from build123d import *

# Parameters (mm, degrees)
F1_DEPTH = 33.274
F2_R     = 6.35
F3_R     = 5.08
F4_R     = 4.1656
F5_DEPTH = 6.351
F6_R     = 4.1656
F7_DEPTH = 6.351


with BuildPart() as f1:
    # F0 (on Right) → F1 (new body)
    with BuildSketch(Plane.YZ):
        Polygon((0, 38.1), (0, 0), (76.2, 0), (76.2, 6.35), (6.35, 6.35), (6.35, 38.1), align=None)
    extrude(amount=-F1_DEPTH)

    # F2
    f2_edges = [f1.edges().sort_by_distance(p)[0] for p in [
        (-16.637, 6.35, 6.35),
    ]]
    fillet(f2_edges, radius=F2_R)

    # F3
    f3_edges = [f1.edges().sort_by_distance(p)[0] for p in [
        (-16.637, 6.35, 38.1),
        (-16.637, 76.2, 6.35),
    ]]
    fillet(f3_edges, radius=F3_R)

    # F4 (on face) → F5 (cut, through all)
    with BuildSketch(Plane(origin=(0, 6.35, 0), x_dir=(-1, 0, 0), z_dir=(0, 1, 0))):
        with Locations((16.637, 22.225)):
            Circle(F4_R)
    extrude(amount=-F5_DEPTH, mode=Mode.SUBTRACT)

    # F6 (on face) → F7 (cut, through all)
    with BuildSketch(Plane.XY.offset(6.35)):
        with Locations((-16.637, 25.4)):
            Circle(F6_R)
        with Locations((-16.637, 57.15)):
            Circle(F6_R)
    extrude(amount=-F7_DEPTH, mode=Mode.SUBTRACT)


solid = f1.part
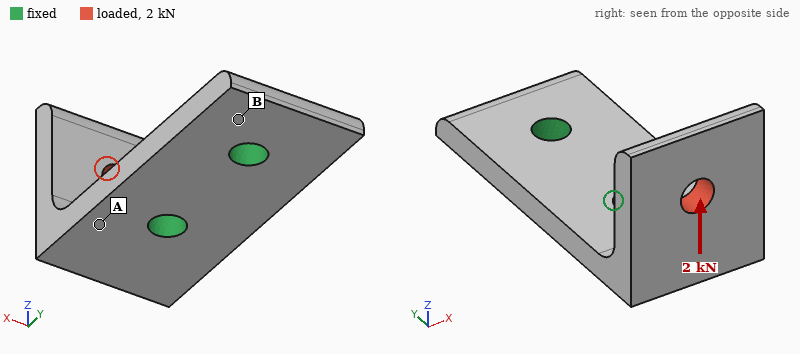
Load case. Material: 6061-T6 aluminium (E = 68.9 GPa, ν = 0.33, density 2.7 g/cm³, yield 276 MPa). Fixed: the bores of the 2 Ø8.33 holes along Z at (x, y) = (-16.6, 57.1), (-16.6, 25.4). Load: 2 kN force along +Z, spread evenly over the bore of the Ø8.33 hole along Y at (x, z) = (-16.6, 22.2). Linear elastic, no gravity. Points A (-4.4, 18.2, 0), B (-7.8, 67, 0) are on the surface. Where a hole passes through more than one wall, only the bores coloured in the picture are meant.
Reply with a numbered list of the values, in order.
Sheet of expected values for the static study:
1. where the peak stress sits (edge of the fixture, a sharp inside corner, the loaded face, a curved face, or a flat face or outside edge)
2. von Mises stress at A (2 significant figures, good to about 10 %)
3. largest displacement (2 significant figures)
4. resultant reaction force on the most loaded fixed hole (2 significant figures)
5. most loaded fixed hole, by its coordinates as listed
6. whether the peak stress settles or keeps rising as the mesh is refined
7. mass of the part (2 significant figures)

1. edge of the fixture
2. 95 MPa
3. 0.34 mm
4. 2.2 kN
5. (-16.6, 25.4)
6. keeps rising
7. 59 g
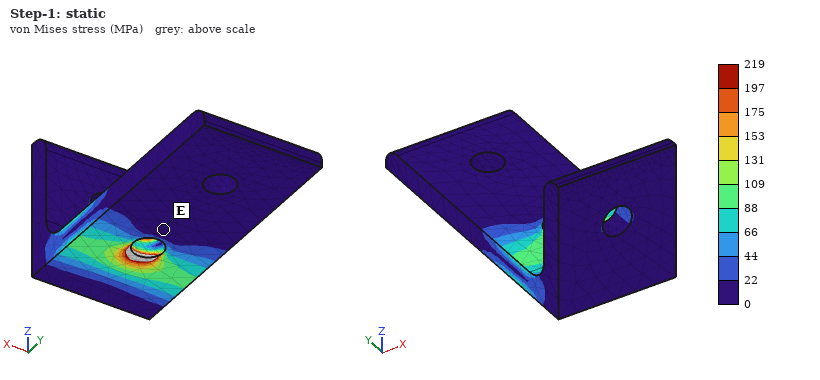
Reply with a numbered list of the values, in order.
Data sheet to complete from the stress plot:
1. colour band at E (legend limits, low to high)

1. 0 to 22 MPa
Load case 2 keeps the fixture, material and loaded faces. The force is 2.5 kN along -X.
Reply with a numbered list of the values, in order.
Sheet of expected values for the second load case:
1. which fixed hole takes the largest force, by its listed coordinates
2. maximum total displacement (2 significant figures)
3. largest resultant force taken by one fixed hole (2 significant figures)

1. (-16.6, 25.4)
2. 0.39 mm
3. 3.5 kN
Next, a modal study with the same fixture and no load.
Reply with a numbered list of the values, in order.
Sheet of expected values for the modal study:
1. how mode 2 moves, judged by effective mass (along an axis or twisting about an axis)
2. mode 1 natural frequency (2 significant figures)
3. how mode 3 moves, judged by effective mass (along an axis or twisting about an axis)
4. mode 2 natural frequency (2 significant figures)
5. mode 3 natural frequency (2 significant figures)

1. along X
2. 2500 Hz
3. along Z
4. 3500 Hz
5. 7400 Hz
